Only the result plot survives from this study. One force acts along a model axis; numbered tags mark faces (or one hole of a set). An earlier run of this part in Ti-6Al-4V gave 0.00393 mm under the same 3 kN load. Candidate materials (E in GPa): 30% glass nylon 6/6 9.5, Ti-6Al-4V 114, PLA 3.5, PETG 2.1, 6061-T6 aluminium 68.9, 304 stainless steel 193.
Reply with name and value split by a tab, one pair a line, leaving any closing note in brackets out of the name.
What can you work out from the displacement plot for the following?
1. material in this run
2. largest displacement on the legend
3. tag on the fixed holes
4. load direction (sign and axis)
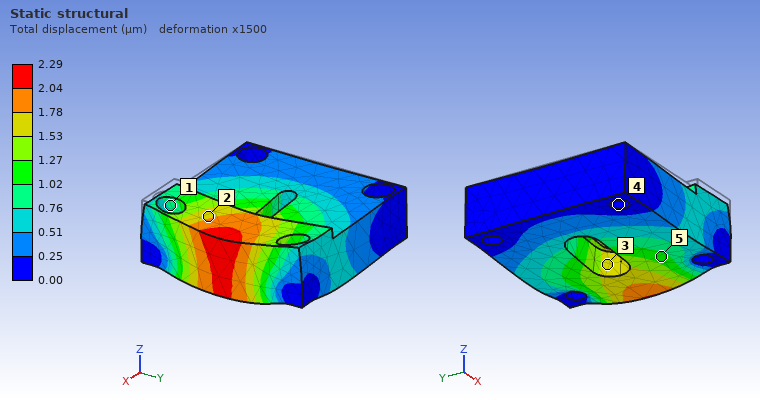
material in this run	304 stainless steel
largest displacement on the legend	2.29 µm
tag on the fixed holes	4
load direction	-Z
